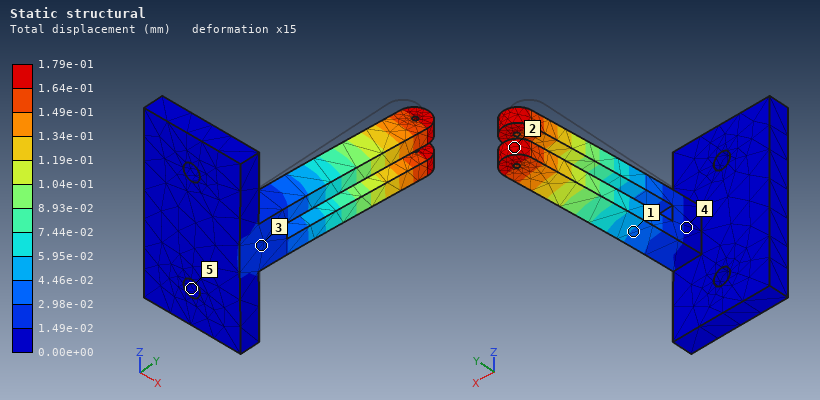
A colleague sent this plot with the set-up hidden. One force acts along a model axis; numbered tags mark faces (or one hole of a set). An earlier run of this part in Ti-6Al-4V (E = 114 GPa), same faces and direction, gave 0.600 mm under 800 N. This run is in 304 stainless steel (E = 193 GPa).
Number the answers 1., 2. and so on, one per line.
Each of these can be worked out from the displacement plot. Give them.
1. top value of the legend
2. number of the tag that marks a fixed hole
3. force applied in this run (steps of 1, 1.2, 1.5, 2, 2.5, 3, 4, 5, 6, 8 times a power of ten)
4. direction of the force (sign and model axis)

1. 1.79e-01 mm
2. 5
3. 400 N
4. +X
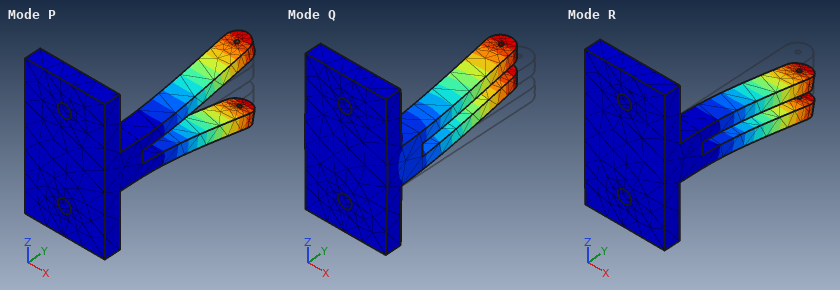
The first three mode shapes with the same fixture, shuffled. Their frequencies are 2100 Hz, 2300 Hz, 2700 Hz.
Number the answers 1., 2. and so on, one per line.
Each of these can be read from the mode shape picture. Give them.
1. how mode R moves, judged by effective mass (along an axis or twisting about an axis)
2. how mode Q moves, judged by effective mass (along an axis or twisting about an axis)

1. along Z
2. along X
